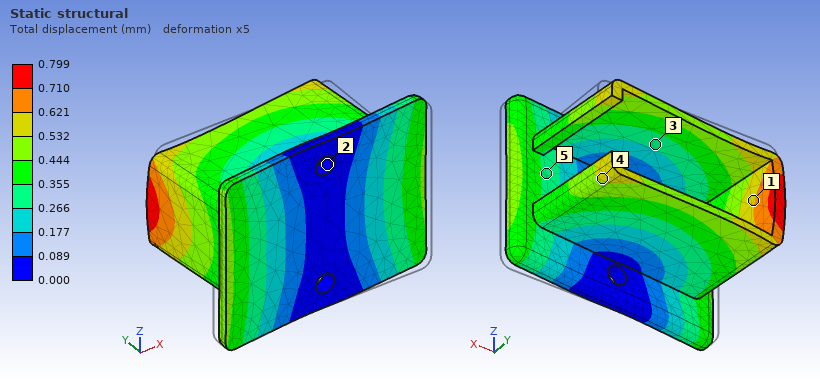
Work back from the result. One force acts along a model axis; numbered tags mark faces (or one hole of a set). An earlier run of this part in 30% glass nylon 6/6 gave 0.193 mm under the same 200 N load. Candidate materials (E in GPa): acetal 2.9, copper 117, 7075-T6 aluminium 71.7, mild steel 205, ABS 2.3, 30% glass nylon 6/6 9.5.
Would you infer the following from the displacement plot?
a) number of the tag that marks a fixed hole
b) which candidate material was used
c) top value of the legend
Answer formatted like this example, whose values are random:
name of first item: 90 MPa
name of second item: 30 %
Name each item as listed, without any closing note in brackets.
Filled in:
number of the tag that marks a fixed hole: 2
which candidate material was used: ABS
top value of the legend: 0.799 mm
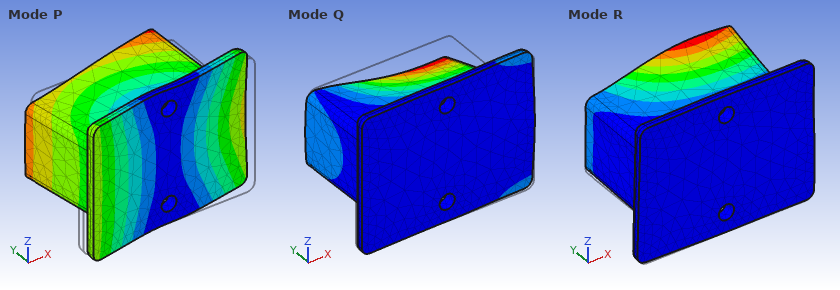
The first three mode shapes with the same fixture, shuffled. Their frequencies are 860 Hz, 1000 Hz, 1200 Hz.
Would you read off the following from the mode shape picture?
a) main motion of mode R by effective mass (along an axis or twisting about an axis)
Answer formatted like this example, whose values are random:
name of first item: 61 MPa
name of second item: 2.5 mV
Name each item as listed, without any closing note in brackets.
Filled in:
main motion of mode R by effective mass: along Z
